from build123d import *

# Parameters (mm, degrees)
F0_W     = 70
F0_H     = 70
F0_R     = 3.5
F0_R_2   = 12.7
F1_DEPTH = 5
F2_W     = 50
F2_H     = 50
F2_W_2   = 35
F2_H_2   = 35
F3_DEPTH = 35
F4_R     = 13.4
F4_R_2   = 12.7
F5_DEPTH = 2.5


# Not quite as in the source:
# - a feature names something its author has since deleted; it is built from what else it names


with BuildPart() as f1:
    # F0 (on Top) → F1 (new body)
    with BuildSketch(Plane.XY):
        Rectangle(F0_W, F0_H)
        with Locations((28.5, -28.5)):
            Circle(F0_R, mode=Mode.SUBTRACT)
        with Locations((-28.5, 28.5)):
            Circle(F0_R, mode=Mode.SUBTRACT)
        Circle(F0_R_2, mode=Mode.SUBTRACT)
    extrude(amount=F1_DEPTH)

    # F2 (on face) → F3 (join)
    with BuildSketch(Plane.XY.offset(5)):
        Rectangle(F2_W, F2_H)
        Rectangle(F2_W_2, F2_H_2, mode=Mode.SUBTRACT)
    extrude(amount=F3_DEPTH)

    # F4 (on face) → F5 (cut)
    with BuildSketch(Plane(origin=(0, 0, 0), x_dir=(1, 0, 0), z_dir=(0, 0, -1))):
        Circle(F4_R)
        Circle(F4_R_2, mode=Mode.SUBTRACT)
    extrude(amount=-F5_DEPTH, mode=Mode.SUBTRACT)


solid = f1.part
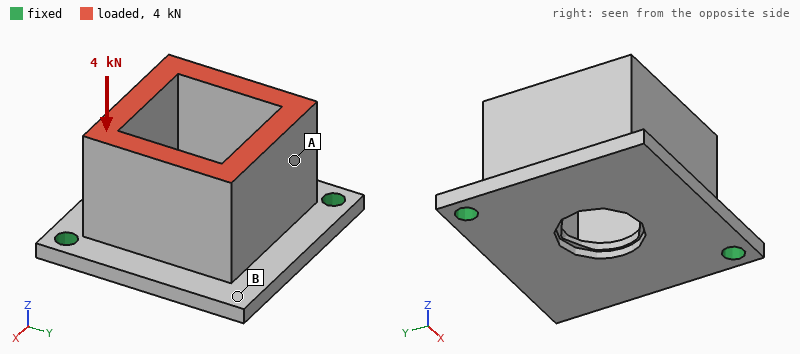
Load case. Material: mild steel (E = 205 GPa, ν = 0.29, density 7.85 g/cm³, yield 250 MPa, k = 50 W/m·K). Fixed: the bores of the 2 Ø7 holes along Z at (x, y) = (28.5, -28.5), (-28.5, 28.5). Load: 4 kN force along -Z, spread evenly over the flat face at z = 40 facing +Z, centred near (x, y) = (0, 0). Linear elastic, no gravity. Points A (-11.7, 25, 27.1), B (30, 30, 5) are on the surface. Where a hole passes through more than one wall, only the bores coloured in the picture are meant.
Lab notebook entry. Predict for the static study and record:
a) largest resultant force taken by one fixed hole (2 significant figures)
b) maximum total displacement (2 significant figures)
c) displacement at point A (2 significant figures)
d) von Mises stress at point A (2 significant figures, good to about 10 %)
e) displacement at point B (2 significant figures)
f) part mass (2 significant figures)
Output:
2.2 kN
19 µm
9.4 µm
18 MPa
18 µm
520 g
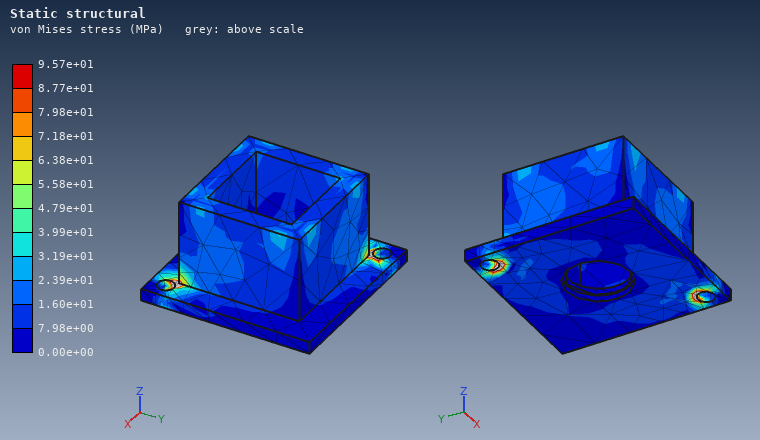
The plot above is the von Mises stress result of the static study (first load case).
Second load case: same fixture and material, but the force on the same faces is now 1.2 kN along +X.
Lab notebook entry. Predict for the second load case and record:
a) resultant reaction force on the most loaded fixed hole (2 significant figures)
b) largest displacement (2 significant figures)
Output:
750 N
86 µm
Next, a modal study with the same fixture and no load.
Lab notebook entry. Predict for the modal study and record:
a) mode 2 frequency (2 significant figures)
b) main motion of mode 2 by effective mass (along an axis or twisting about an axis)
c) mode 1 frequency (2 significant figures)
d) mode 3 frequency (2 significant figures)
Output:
3800 Hz
along Z
1200 Hz
7400 Hz
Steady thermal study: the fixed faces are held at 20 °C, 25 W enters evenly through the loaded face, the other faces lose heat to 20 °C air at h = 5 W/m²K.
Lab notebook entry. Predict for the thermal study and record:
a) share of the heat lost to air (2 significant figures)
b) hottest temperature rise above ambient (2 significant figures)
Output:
11 %
38 K
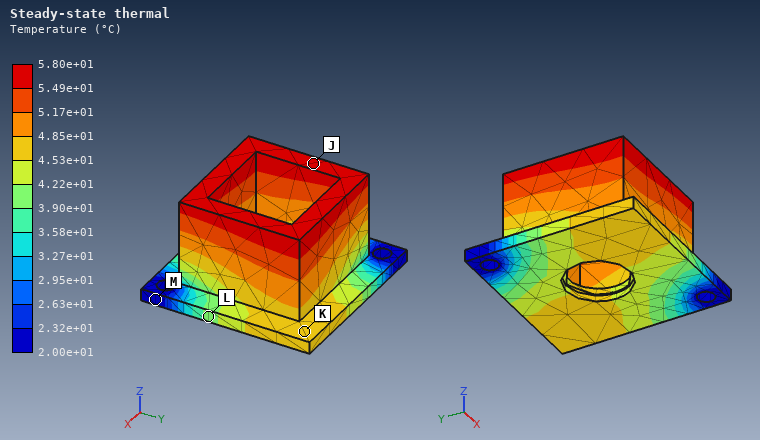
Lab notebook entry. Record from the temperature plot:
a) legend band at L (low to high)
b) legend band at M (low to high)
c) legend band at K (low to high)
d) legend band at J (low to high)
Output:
3.90e+01 to 4.22e+01 °C
2.00e+01 to 2.32e+01 °C
4.53e+01 to 4.85e+01 °C
5.49e+01 to 5.80e+01 °C
